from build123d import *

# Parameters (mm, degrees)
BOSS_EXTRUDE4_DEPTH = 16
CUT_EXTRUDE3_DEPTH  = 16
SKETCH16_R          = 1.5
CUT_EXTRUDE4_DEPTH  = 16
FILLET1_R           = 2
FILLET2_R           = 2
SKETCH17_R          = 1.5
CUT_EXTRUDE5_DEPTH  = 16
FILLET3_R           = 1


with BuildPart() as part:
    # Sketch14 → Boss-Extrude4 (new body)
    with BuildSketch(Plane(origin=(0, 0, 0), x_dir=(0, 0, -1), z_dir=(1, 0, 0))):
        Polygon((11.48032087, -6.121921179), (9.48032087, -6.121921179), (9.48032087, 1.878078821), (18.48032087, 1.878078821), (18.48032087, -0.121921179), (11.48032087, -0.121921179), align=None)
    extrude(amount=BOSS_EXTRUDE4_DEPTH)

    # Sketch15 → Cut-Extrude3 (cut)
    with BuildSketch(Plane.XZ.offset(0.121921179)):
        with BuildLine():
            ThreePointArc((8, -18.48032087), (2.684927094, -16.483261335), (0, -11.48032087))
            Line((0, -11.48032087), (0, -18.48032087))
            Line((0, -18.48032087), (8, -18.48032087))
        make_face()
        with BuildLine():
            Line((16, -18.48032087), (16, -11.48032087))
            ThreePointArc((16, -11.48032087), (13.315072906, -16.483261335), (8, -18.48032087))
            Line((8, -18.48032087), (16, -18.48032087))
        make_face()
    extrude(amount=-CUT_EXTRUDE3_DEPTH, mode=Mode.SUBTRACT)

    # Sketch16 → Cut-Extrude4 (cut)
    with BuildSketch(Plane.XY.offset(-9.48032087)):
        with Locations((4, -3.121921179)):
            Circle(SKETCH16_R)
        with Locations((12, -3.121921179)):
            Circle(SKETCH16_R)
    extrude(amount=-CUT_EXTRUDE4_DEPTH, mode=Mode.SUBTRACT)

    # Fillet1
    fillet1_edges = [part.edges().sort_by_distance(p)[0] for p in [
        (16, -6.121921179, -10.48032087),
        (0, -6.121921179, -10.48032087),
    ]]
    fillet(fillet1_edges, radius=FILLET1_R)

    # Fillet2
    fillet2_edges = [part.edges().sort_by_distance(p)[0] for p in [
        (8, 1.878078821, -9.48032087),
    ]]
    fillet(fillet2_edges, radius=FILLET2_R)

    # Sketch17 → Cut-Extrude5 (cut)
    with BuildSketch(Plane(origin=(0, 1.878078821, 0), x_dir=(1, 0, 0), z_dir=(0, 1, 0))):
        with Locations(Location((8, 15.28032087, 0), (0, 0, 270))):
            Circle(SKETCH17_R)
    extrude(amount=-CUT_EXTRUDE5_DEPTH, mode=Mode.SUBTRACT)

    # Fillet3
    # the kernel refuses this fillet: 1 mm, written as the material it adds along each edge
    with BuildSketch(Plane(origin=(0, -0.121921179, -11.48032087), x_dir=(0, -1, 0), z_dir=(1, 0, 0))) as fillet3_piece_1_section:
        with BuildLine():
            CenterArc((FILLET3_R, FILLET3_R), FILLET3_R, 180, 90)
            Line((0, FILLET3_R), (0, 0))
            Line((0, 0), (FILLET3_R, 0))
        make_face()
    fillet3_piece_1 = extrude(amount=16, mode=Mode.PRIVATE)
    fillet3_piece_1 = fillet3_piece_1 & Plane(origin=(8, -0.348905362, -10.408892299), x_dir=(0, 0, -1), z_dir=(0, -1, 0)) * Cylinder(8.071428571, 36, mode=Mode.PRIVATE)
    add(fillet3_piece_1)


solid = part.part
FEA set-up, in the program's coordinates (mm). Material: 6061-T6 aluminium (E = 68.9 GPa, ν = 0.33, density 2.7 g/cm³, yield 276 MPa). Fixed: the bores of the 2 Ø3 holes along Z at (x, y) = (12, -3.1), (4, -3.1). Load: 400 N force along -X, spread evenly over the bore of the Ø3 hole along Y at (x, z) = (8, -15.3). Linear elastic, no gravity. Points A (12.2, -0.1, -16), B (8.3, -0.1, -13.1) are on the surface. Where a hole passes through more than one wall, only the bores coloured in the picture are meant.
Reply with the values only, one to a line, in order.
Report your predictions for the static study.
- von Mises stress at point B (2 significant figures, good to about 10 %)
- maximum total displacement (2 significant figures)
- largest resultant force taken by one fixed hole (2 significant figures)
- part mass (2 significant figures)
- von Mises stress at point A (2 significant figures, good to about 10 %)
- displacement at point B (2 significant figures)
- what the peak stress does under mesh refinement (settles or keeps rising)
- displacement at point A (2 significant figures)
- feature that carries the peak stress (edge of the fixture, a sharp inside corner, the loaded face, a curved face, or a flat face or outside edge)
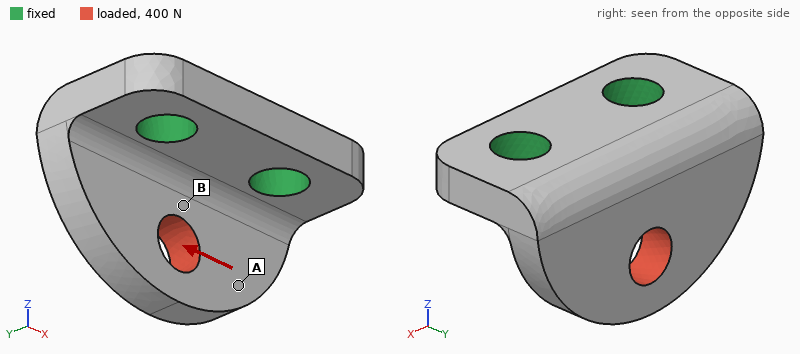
77 MPa
15 µm
300 N
1.00 g
26 MPa
5.7 µm
keeps rising
12 µm
edge of the fixture
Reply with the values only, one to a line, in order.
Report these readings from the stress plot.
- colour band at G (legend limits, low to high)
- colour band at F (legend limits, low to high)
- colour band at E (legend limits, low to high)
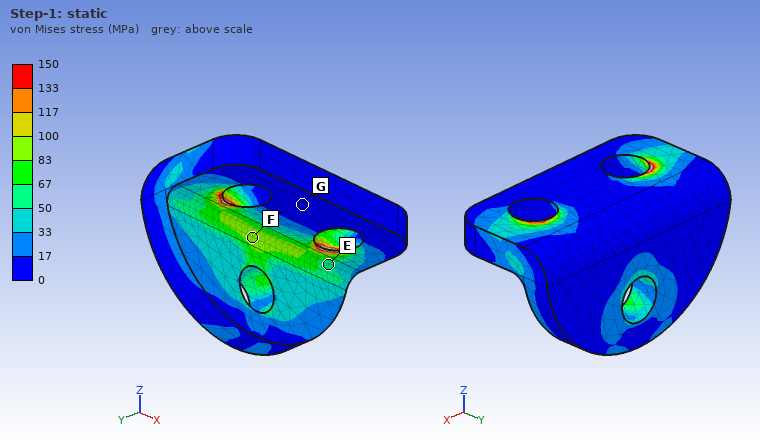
0 to 17 MPa
83 to 100 MPa
50 to 67 MPa
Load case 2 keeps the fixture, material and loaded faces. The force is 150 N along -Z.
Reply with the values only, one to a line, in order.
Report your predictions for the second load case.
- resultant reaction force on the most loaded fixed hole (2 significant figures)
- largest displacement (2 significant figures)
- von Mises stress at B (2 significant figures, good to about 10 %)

76 N
9.9 µm
7.4 MPa
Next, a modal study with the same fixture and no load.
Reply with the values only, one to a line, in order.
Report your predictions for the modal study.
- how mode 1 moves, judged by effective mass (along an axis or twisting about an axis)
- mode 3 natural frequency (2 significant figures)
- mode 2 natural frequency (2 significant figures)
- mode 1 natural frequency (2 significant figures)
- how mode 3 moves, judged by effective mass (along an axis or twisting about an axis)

along Y
62 kHz
40 kHz
23 kHz
along X
